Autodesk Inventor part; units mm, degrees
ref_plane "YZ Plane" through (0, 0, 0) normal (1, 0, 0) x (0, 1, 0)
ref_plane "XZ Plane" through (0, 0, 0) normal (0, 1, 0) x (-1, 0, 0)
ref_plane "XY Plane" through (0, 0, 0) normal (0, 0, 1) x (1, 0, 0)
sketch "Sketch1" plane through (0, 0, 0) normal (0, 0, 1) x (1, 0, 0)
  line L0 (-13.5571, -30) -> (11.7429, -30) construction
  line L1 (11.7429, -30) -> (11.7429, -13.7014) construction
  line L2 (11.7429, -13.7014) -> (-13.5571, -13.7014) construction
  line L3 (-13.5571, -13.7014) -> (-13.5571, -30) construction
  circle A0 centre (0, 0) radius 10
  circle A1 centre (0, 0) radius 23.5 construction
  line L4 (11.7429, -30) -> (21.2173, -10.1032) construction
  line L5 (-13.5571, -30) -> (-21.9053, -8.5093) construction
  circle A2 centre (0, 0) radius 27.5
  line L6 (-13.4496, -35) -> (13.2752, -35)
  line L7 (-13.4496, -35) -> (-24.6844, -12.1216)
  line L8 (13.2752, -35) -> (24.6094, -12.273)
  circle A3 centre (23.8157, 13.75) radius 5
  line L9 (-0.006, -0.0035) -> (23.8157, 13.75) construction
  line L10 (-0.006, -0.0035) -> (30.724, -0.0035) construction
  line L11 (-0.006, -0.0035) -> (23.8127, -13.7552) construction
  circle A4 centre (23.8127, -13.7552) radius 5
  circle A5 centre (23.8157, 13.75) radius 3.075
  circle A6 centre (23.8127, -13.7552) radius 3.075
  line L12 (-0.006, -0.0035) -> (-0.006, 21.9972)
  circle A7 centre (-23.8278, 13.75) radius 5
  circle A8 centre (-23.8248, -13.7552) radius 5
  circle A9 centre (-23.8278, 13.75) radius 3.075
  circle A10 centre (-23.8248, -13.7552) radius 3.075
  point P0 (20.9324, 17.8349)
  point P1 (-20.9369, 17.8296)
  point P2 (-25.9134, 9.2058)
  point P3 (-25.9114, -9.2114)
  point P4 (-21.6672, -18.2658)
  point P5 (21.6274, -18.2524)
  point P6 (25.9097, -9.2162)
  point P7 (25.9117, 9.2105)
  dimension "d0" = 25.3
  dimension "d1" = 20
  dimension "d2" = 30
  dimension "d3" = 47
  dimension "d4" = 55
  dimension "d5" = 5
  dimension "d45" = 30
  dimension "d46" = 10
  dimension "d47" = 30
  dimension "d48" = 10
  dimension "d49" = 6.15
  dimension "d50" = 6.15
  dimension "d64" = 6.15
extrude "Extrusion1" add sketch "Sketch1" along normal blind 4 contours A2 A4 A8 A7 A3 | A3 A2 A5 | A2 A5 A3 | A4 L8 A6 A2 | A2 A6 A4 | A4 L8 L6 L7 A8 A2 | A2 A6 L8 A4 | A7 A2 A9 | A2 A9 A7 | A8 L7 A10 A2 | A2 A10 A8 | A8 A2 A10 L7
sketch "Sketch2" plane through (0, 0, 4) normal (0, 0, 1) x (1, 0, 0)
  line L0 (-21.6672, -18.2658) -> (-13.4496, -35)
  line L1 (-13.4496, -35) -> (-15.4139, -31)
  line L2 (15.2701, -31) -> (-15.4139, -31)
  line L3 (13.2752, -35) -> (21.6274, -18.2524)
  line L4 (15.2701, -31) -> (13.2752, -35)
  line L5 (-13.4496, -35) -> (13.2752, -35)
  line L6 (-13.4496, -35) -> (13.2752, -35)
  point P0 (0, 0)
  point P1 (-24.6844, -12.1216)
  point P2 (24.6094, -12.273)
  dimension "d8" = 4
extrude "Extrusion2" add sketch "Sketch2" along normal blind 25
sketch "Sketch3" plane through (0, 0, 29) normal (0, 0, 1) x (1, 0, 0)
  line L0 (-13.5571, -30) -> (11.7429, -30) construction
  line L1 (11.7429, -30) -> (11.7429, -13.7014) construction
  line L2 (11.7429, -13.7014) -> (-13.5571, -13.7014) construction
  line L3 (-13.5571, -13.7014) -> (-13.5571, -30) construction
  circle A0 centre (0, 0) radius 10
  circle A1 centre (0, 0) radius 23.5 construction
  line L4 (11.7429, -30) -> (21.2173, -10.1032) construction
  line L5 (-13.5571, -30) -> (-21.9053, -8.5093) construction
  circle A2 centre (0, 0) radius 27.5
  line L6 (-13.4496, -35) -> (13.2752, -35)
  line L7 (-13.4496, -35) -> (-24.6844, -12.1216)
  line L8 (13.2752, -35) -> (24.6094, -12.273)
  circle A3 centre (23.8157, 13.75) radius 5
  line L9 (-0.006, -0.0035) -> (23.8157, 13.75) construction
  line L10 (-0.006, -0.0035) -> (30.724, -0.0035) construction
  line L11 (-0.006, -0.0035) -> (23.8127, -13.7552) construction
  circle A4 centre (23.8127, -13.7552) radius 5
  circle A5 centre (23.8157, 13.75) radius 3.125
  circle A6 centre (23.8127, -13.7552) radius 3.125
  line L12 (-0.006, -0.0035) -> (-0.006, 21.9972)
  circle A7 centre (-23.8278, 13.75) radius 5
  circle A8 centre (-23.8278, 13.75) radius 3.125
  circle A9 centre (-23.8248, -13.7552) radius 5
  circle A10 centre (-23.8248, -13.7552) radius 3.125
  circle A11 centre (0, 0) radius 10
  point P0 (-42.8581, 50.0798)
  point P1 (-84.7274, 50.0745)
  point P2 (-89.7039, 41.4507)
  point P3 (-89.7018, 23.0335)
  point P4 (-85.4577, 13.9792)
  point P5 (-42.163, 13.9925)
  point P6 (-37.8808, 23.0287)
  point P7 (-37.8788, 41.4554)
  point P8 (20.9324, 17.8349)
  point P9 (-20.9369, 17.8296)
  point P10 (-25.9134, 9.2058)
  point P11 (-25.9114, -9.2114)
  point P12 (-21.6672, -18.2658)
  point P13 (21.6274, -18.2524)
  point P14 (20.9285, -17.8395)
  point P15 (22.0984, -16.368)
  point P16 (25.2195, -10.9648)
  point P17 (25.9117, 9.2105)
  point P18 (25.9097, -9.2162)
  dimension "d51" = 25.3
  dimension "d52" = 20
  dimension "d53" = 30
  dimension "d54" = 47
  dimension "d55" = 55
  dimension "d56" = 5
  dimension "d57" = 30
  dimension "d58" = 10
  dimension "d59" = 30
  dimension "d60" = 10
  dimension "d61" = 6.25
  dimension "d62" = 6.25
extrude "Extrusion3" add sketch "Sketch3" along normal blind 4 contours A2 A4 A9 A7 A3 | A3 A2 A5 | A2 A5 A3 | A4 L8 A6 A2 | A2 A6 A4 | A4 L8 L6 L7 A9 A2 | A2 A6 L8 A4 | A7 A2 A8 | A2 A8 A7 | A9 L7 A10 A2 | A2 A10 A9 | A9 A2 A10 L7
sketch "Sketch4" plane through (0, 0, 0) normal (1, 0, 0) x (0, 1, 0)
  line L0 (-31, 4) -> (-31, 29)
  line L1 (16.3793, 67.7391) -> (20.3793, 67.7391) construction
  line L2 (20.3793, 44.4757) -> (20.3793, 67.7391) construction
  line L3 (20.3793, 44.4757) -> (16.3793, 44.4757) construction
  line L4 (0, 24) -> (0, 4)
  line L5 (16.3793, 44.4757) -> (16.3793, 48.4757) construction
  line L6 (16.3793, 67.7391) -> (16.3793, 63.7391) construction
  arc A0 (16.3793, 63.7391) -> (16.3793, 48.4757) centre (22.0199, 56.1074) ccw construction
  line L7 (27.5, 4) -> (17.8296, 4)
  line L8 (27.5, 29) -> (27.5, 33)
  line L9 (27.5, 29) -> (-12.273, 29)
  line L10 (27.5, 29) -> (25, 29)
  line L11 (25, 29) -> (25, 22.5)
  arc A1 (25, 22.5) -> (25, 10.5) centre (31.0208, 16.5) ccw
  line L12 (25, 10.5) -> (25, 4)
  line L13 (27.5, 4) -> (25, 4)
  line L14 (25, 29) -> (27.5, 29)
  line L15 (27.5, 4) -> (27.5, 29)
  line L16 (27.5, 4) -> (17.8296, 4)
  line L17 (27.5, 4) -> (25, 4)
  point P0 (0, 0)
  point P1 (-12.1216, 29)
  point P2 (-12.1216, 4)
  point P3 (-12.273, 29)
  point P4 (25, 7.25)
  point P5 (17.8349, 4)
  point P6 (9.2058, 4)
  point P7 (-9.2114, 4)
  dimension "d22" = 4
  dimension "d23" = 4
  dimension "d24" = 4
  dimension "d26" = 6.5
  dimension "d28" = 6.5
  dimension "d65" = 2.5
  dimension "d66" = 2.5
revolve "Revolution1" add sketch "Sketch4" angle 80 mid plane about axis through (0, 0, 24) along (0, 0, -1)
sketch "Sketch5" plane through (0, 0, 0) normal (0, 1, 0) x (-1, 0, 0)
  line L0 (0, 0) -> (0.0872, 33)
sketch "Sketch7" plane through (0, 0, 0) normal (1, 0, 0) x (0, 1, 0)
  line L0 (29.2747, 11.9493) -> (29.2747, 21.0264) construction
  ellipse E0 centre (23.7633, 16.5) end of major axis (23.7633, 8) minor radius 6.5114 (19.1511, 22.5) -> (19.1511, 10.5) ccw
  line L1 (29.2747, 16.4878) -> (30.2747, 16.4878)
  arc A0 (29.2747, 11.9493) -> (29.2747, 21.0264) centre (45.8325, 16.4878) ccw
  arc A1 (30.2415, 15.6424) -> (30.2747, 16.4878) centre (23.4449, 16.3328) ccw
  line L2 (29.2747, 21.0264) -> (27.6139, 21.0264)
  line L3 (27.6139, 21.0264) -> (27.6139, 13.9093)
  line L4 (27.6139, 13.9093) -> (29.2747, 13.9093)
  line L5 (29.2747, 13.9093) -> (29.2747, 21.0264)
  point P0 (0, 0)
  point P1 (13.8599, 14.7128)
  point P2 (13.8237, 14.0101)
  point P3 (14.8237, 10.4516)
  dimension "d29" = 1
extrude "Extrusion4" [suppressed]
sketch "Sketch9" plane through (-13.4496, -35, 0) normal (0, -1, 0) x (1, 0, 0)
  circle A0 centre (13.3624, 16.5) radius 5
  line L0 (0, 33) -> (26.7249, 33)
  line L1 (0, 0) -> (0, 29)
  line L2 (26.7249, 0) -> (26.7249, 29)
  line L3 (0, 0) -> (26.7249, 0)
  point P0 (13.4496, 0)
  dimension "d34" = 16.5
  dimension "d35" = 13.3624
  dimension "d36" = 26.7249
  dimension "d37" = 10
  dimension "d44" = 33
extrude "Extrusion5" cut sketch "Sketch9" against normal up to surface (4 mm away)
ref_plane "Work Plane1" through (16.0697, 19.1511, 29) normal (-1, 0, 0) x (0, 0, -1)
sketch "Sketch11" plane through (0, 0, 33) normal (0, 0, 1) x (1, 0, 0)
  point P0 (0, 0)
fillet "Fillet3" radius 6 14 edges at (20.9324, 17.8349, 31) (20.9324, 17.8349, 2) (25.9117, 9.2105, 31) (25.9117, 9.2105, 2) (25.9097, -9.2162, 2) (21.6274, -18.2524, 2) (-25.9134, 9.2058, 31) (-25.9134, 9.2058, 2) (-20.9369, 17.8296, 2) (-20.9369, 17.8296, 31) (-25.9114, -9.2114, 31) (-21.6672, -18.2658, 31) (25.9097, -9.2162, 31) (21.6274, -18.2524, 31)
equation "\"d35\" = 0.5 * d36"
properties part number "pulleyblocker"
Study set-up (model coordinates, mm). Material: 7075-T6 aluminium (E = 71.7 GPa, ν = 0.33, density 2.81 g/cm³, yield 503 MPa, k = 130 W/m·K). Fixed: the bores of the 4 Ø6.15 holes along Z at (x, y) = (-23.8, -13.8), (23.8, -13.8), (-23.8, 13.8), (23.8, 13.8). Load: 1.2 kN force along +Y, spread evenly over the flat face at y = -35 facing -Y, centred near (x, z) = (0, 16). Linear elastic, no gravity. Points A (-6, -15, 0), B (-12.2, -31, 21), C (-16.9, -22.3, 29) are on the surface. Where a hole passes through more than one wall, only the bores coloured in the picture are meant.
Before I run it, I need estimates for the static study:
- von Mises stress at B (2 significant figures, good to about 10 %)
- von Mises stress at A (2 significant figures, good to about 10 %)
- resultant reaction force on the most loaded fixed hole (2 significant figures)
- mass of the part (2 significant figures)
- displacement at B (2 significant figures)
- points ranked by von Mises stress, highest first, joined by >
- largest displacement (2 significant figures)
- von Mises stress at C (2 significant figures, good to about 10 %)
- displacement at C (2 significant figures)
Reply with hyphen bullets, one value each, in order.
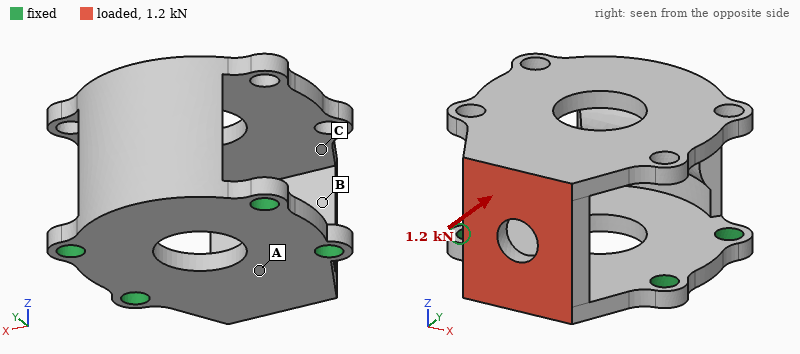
- 58 MPa
- 35 MPa
- 430 N
- 70 g
- 0.22 mm
- B > A > C
- 0.30 mm
- 15 MPa
- 0.27 mm
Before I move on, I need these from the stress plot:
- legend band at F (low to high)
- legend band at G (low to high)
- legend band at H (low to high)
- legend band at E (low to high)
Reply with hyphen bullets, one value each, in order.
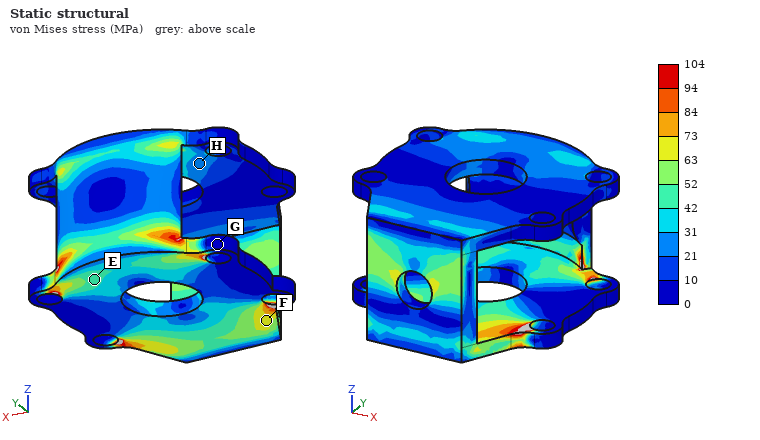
- 63 to 73 MPa
- 0 to 10 MPa
- 21 to 31 MPa
- 42 to 52 MPa
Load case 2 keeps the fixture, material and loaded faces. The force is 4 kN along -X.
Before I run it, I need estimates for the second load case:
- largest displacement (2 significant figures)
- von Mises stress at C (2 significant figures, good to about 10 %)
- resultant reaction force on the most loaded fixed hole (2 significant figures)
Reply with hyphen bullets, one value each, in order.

- 0.63 mm
- 63 MPa
- 2.8 kN
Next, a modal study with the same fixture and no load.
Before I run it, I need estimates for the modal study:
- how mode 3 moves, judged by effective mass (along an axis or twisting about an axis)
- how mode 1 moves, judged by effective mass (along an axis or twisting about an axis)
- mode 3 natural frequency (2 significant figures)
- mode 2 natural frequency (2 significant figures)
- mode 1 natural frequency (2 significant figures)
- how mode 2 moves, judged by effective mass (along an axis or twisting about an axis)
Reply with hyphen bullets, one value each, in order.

- along Z
- along Y
- 2600 Hz
- 2300 Hz
- 1300 Hz
- along X
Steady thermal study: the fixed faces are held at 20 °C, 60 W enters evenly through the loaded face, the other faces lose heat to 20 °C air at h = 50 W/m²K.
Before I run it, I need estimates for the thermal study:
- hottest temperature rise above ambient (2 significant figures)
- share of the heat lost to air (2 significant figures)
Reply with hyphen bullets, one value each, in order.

- 71 K
- 33 %
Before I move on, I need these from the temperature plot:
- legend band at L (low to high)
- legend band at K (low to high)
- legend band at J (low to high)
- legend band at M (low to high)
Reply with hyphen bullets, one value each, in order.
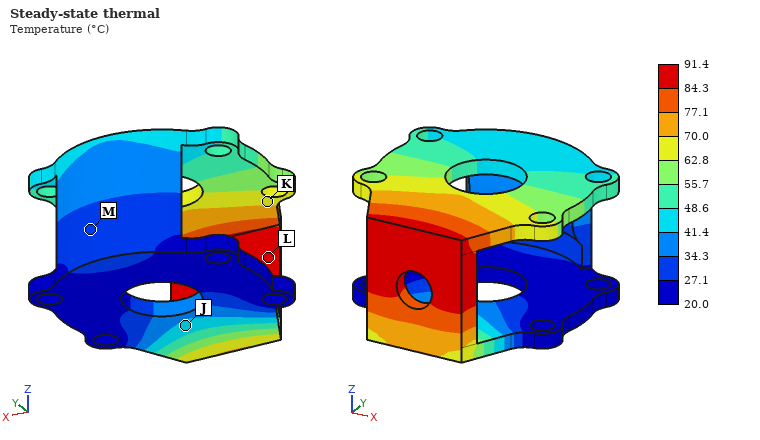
- 84.3 to 91.4 °C
- 62.8 to 70.0 °C
- 41.4 to 48.6 °C
- 27.1 to 34.3 °C
